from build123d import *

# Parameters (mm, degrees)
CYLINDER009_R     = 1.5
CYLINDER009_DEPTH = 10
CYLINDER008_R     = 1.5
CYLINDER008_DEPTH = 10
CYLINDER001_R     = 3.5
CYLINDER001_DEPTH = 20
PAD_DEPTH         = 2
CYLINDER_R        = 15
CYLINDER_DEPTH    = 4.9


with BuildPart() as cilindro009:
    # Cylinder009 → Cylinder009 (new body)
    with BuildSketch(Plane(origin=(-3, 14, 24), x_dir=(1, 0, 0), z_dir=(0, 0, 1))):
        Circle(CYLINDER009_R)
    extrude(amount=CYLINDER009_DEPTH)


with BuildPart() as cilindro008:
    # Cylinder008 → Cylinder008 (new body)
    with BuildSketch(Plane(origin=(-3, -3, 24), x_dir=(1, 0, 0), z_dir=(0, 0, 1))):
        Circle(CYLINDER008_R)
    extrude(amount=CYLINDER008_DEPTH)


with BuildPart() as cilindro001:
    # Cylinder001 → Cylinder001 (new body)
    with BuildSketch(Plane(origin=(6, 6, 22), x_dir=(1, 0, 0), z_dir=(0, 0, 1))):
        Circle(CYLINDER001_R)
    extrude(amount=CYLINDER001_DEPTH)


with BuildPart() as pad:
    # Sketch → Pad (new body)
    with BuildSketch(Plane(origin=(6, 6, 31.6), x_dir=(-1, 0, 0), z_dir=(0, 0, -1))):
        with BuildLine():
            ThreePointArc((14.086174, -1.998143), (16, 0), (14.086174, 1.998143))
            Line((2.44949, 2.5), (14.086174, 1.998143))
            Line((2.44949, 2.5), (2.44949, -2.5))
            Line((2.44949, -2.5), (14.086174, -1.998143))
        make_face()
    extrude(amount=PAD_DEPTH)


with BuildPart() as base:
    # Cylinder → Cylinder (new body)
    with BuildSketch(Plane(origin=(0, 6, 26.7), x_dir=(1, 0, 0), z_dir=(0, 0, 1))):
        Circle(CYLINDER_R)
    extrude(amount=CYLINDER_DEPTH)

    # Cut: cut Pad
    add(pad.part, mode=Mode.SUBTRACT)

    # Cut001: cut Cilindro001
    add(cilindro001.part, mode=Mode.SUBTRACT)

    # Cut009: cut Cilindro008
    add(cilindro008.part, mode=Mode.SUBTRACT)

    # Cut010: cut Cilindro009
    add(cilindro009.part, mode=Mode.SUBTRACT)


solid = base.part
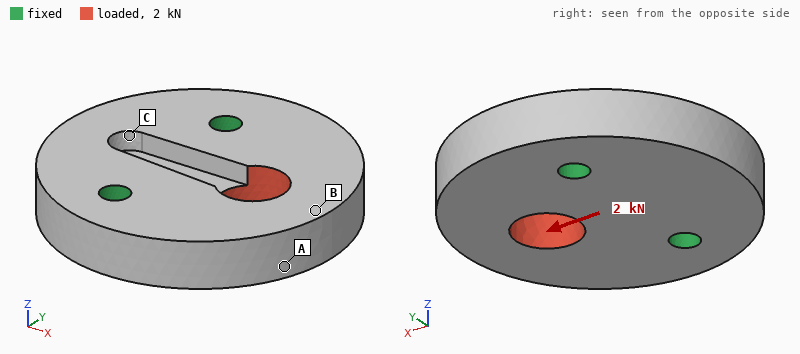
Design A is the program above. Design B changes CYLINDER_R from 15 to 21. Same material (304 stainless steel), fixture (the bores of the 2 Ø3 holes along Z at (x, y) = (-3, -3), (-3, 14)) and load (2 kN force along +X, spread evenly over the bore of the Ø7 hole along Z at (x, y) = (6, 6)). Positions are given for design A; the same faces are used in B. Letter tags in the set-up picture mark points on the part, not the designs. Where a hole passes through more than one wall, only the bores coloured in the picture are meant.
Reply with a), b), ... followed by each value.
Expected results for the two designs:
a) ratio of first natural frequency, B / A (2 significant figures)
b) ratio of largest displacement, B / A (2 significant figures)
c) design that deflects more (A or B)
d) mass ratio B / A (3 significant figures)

a) 0.54
b) 0.78
c) A
d) 2.07
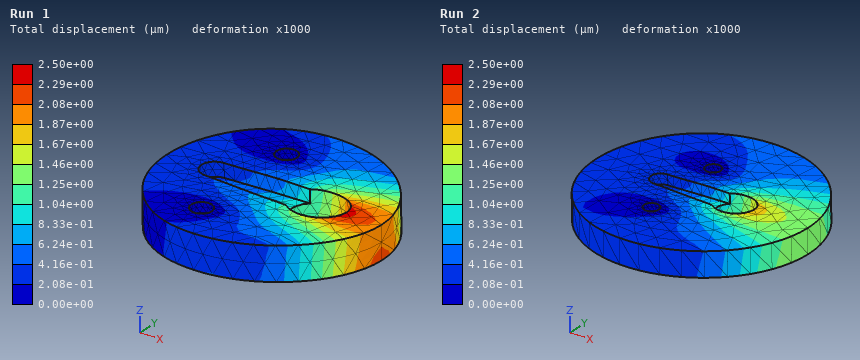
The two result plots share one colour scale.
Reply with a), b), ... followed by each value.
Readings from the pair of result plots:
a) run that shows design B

a) Run 2
